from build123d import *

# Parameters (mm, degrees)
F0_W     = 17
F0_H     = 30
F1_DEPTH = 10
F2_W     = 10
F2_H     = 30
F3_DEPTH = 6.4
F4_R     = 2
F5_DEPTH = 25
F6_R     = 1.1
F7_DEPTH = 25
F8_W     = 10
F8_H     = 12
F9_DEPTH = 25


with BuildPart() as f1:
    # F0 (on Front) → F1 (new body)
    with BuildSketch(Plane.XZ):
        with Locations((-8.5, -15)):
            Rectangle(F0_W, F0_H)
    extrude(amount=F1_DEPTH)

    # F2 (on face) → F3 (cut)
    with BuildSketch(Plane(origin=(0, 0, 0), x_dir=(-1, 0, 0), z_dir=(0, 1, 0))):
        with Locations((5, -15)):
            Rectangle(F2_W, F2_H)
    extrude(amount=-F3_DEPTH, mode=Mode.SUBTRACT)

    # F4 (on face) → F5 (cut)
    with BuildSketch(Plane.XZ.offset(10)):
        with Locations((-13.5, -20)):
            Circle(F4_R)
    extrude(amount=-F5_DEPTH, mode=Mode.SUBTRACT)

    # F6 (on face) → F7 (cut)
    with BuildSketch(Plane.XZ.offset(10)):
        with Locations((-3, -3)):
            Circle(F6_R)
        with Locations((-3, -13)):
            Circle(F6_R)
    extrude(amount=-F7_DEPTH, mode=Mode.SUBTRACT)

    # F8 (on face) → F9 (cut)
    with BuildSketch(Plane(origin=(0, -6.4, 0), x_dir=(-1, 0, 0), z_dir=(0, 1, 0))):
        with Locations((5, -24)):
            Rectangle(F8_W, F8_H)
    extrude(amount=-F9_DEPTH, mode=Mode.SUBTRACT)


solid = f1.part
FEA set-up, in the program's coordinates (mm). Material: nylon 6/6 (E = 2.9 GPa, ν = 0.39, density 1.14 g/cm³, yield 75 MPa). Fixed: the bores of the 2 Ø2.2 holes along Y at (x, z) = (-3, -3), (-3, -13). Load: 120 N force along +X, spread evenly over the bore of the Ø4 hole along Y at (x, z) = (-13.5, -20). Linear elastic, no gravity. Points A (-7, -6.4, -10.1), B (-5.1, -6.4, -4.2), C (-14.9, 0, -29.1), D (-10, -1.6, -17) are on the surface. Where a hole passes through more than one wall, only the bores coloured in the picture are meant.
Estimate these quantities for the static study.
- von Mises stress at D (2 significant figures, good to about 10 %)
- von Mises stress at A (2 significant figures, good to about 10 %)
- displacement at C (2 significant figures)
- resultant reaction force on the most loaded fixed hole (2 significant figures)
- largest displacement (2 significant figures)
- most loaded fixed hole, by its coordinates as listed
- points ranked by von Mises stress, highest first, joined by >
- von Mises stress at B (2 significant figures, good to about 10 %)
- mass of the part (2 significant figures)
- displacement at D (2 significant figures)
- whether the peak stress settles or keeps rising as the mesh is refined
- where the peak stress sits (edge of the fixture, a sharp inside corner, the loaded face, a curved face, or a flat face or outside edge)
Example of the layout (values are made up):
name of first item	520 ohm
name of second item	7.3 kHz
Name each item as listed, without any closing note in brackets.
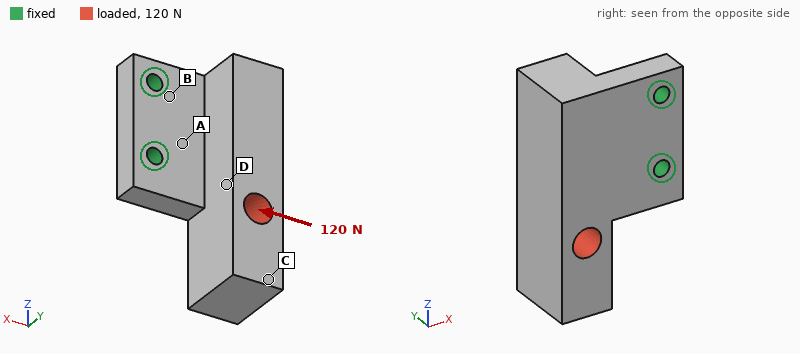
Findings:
von Mises stress at D	4.6 MPa
von Mises stress at A	11 MPa
displacement at C	0.34 mm
resultant reaction force on the most loaded fixed hole	190 N
largest displacement	0.37 mm
most loaded fixed hole, by its coordinates as listed	(-3, -13)
points ranked by von Mises stress, highest first, joined by >	A > B > D > C
von Mises stress at B	7.6 MPa
mass of the part	3.0 g
displacement at D	0.17 mm
whether the peak stress settles or keeps rising as the mesh is refined	keeps rising
where the peak stress sits	edge of the fixture
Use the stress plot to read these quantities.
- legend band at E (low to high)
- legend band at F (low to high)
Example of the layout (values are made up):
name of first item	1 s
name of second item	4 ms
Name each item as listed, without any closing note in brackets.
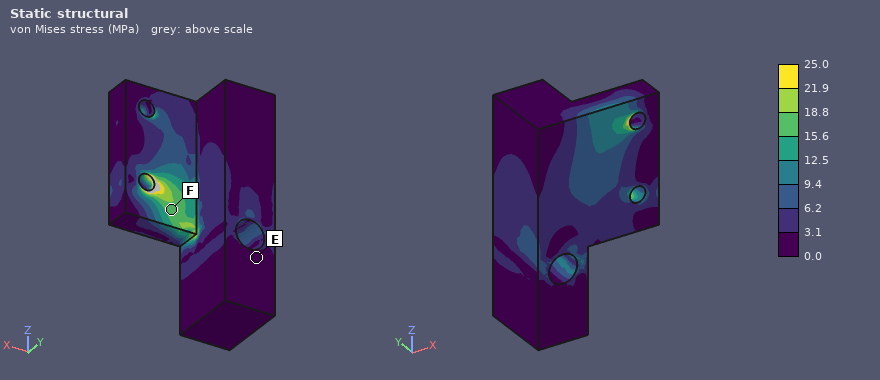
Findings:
legend band at E	0.0 to 3.1 MPa
legend band at F	15.6 to 18.8 MPa
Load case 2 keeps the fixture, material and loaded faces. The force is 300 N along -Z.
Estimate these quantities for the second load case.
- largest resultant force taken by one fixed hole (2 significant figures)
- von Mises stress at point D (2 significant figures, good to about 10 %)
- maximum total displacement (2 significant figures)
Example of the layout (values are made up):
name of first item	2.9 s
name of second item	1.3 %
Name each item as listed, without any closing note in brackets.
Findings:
largest resultant force taken by one fixed hole	320 N
von Mises stress at point D	4.5 MPa
maximum total displacement	0.35 mm
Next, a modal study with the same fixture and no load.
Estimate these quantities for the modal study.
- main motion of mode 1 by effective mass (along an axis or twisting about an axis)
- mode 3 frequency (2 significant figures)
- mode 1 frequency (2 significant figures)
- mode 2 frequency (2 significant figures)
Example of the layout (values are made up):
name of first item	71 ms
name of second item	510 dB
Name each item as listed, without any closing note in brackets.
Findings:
main motion of mode 1 by effective mass	along Y
mode 3 frequency	3900 Hz
mode 1 frequency	1700 Hz
mode 2 frequency	3000 Hz
